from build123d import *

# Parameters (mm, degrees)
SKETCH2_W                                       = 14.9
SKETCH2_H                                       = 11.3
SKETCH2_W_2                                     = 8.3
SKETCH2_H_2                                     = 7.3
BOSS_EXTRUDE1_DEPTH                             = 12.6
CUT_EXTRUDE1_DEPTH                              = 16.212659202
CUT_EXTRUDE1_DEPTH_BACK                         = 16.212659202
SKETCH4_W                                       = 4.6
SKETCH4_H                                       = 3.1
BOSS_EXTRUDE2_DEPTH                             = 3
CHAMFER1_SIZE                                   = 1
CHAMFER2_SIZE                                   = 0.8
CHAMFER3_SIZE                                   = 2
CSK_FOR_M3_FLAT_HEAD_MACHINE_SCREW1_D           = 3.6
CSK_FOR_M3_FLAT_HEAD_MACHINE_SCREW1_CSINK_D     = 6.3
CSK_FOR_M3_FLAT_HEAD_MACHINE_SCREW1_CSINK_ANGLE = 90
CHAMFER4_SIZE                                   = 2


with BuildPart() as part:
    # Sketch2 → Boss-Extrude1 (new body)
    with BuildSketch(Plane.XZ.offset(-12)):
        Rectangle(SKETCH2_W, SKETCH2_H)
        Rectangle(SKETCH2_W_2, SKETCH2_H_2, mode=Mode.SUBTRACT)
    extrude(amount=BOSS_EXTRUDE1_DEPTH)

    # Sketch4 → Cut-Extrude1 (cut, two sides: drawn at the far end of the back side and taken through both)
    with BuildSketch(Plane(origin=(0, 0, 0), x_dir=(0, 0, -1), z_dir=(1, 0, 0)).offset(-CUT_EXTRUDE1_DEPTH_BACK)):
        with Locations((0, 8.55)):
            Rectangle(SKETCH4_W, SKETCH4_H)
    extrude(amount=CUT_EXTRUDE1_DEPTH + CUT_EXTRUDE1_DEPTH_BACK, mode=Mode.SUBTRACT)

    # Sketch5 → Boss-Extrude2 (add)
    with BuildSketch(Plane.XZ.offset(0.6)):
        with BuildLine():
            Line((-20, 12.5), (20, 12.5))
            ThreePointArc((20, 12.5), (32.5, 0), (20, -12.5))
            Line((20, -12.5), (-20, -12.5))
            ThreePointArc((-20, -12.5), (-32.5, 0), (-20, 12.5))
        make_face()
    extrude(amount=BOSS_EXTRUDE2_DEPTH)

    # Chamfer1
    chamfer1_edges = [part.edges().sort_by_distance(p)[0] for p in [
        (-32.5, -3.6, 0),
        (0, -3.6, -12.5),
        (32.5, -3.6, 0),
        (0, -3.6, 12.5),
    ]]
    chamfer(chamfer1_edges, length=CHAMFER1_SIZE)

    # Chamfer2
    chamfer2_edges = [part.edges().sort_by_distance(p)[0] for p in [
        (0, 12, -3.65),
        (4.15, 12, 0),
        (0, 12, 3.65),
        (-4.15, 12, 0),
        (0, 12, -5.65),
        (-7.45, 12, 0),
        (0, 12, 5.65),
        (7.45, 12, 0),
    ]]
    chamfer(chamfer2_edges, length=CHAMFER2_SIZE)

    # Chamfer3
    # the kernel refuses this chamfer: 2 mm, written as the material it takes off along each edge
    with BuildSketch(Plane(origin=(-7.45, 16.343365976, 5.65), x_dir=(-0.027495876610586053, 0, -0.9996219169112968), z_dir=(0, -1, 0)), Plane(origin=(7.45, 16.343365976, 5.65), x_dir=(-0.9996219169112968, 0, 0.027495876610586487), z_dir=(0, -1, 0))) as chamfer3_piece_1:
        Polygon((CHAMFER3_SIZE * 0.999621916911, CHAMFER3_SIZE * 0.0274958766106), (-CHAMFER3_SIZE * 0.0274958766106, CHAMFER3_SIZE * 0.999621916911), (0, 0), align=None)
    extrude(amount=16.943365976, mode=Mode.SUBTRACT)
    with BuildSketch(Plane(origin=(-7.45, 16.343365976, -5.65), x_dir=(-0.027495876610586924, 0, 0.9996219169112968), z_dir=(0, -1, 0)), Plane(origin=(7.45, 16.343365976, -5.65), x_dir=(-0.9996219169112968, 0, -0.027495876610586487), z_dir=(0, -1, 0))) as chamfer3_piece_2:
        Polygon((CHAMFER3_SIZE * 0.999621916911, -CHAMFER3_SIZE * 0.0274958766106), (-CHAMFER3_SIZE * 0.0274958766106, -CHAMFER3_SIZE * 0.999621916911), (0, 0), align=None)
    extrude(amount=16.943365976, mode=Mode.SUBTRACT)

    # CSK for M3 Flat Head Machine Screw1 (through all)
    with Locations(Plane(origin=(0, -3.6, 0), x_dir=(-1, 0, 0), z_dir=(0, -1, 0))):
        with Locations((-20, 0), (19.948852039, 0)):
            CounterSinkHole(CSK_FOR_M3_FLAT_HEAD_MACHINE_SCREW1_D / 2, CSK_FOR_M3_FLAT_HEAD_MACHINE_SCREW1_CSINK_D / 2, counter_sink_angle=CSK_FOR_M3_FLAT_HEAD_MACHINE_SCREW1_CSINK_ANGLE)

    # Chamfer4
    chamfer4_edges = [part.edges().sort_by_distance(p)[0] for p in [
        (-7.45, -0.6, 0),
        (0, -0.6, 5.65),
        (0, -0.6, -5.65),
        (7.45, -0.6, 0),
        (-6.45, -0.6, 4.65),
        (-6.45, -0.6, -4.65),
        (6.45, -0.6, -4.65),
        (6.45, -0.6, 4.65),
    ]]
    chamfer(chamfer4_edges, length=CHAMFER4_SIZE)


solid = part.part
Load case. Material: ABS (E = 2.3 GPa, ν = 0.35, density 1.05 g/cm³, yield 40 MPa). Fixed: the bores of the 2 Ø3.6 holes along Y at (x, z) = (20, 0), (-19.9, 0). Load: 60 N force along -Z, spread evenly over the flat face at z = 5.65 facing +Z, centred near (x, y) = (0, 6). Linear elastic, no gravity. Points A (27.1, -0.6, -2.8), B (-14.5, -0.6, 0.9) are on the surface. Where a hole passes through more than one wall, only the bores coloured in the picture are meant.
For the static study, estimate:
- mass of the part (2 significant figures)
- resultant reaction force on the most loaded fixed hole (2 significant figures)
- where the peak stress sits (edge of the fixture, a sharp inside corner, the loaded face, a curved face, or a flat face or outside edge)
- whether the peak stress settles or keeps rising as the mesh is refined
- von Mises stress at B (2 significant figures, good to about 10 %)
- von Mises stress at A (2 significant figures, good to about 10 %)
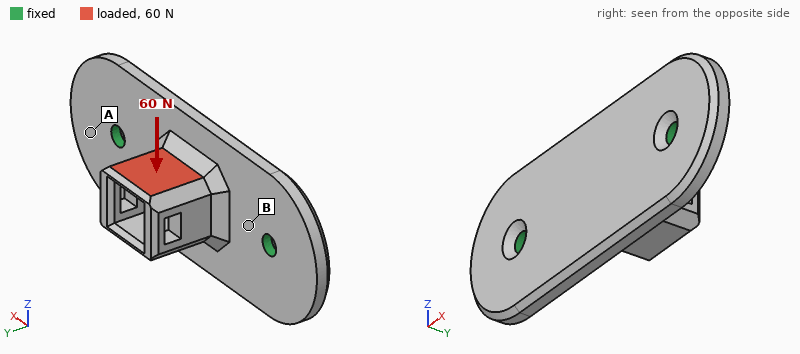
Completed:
5.8 g
30 N
edge of the fixture
keeps rising
6.5 MPa
1.5 MPa
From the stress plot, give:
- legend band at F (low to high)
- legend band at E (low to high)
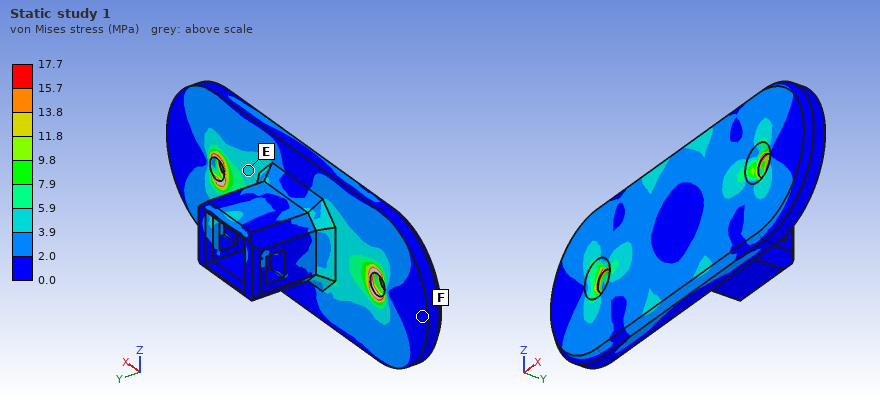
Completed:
0.0 to 2.0 MPa
3.9 to 5.9 MPa
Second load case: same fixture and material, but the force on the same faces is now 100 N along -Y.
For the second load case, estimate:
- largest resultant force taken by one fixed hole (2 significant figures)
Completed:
52 N
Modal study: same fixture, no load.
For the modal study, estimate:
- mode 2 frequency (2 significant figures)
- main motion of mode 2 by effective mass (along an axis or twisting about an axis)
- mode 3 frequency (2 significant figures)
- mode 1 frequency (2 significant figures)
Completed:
2100 Hz
along Y
3900 Hz
1600 Hz
